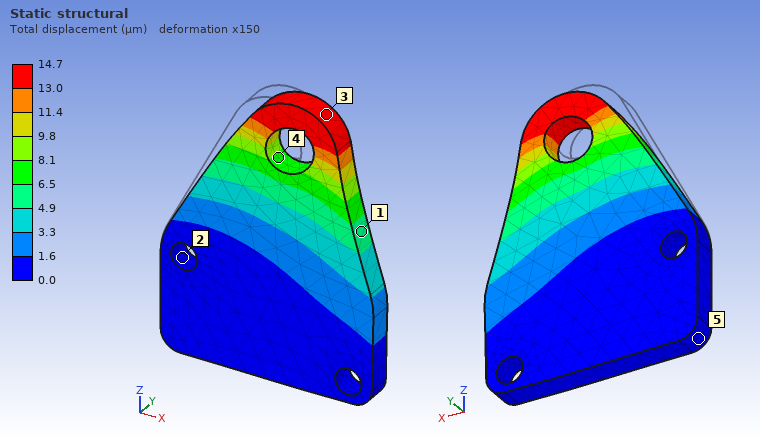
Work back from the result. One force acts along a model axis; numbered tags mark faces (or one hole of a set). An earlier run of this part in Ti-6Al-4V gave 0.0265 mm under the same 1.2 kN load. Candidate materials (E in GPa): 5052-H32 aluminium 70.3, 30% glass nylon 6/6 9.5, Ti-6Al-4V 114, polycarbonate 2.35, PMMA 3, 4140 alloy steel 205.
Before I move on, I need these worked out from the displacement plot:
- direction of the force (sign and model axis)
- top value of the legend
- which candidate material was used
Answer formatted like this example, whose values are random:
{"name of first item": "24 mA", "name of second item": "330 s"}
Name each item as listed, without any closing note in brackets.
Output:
{"direction of the force": "+X", "top value of the legend": "14.7 µm", "which candidate material was used": "4140 alloy steel"}
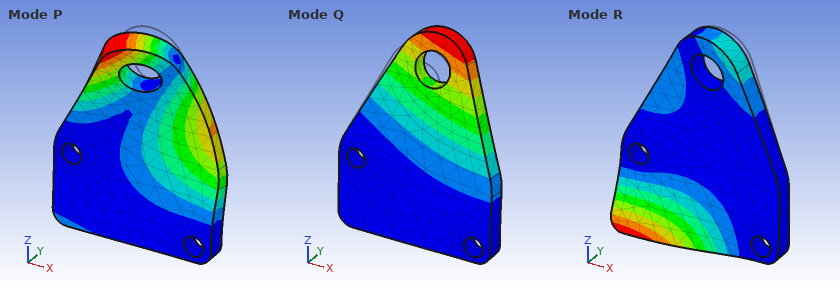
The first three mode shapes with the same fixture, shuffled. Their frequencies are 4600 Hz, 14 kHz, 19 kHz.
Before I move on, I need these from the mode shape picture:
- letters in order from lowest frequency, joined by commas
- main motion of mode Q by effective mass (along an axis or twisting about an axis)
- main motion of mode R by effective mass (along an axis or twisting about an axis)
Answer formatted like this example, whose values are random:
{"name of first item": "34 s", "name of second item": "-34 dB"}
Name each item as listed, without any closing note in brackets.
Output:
{"letters in order from lowest frequency, joined by commas": "Q, P, R", "main motion of mode Q by effective mass": "along Y", "main motion of mode R by effective mass": "along Y"}
